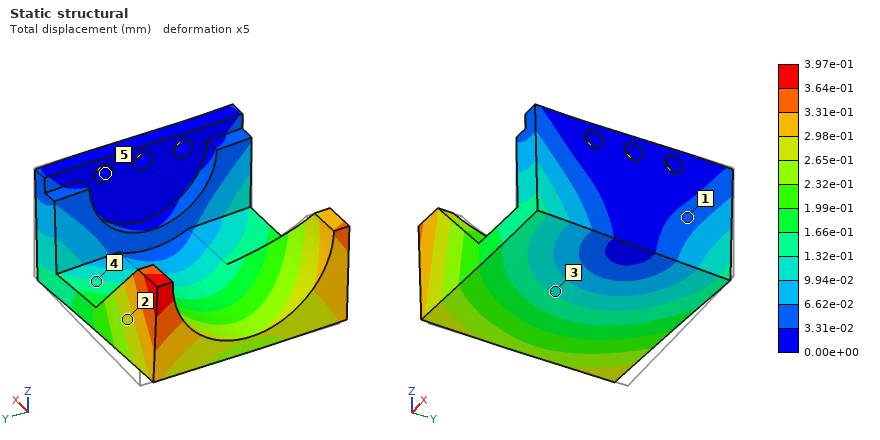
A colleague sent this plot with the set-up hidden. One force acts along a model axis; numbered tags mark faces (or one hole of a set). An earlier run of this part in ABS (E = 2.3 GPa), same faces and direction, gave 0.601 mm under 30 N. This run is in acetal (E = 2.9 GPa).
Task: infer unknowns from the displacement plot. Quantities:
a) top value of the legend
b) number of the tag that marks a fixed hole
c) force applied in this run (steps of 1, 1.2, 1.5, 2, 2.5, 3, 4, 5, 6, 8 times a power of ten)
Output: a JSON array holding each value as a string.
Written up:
["3.97e-01 mm", "5", "25 N"]
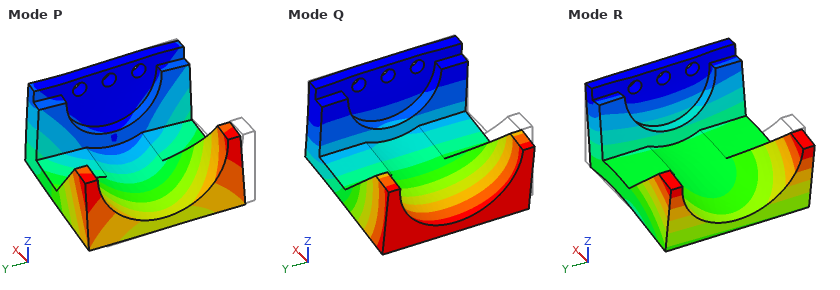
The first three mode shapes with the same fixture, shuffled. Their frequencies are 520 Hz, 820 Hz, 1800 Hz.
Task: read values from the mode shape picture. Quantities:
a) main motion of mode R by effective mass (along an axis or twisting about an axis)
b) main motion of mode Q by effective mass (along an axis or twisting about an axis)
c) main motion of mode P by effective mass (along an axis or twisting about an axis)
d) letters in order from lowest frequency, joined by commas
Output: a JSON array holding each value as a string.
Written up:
["along X", "along Z", "along Y", "Q, P, R"]
